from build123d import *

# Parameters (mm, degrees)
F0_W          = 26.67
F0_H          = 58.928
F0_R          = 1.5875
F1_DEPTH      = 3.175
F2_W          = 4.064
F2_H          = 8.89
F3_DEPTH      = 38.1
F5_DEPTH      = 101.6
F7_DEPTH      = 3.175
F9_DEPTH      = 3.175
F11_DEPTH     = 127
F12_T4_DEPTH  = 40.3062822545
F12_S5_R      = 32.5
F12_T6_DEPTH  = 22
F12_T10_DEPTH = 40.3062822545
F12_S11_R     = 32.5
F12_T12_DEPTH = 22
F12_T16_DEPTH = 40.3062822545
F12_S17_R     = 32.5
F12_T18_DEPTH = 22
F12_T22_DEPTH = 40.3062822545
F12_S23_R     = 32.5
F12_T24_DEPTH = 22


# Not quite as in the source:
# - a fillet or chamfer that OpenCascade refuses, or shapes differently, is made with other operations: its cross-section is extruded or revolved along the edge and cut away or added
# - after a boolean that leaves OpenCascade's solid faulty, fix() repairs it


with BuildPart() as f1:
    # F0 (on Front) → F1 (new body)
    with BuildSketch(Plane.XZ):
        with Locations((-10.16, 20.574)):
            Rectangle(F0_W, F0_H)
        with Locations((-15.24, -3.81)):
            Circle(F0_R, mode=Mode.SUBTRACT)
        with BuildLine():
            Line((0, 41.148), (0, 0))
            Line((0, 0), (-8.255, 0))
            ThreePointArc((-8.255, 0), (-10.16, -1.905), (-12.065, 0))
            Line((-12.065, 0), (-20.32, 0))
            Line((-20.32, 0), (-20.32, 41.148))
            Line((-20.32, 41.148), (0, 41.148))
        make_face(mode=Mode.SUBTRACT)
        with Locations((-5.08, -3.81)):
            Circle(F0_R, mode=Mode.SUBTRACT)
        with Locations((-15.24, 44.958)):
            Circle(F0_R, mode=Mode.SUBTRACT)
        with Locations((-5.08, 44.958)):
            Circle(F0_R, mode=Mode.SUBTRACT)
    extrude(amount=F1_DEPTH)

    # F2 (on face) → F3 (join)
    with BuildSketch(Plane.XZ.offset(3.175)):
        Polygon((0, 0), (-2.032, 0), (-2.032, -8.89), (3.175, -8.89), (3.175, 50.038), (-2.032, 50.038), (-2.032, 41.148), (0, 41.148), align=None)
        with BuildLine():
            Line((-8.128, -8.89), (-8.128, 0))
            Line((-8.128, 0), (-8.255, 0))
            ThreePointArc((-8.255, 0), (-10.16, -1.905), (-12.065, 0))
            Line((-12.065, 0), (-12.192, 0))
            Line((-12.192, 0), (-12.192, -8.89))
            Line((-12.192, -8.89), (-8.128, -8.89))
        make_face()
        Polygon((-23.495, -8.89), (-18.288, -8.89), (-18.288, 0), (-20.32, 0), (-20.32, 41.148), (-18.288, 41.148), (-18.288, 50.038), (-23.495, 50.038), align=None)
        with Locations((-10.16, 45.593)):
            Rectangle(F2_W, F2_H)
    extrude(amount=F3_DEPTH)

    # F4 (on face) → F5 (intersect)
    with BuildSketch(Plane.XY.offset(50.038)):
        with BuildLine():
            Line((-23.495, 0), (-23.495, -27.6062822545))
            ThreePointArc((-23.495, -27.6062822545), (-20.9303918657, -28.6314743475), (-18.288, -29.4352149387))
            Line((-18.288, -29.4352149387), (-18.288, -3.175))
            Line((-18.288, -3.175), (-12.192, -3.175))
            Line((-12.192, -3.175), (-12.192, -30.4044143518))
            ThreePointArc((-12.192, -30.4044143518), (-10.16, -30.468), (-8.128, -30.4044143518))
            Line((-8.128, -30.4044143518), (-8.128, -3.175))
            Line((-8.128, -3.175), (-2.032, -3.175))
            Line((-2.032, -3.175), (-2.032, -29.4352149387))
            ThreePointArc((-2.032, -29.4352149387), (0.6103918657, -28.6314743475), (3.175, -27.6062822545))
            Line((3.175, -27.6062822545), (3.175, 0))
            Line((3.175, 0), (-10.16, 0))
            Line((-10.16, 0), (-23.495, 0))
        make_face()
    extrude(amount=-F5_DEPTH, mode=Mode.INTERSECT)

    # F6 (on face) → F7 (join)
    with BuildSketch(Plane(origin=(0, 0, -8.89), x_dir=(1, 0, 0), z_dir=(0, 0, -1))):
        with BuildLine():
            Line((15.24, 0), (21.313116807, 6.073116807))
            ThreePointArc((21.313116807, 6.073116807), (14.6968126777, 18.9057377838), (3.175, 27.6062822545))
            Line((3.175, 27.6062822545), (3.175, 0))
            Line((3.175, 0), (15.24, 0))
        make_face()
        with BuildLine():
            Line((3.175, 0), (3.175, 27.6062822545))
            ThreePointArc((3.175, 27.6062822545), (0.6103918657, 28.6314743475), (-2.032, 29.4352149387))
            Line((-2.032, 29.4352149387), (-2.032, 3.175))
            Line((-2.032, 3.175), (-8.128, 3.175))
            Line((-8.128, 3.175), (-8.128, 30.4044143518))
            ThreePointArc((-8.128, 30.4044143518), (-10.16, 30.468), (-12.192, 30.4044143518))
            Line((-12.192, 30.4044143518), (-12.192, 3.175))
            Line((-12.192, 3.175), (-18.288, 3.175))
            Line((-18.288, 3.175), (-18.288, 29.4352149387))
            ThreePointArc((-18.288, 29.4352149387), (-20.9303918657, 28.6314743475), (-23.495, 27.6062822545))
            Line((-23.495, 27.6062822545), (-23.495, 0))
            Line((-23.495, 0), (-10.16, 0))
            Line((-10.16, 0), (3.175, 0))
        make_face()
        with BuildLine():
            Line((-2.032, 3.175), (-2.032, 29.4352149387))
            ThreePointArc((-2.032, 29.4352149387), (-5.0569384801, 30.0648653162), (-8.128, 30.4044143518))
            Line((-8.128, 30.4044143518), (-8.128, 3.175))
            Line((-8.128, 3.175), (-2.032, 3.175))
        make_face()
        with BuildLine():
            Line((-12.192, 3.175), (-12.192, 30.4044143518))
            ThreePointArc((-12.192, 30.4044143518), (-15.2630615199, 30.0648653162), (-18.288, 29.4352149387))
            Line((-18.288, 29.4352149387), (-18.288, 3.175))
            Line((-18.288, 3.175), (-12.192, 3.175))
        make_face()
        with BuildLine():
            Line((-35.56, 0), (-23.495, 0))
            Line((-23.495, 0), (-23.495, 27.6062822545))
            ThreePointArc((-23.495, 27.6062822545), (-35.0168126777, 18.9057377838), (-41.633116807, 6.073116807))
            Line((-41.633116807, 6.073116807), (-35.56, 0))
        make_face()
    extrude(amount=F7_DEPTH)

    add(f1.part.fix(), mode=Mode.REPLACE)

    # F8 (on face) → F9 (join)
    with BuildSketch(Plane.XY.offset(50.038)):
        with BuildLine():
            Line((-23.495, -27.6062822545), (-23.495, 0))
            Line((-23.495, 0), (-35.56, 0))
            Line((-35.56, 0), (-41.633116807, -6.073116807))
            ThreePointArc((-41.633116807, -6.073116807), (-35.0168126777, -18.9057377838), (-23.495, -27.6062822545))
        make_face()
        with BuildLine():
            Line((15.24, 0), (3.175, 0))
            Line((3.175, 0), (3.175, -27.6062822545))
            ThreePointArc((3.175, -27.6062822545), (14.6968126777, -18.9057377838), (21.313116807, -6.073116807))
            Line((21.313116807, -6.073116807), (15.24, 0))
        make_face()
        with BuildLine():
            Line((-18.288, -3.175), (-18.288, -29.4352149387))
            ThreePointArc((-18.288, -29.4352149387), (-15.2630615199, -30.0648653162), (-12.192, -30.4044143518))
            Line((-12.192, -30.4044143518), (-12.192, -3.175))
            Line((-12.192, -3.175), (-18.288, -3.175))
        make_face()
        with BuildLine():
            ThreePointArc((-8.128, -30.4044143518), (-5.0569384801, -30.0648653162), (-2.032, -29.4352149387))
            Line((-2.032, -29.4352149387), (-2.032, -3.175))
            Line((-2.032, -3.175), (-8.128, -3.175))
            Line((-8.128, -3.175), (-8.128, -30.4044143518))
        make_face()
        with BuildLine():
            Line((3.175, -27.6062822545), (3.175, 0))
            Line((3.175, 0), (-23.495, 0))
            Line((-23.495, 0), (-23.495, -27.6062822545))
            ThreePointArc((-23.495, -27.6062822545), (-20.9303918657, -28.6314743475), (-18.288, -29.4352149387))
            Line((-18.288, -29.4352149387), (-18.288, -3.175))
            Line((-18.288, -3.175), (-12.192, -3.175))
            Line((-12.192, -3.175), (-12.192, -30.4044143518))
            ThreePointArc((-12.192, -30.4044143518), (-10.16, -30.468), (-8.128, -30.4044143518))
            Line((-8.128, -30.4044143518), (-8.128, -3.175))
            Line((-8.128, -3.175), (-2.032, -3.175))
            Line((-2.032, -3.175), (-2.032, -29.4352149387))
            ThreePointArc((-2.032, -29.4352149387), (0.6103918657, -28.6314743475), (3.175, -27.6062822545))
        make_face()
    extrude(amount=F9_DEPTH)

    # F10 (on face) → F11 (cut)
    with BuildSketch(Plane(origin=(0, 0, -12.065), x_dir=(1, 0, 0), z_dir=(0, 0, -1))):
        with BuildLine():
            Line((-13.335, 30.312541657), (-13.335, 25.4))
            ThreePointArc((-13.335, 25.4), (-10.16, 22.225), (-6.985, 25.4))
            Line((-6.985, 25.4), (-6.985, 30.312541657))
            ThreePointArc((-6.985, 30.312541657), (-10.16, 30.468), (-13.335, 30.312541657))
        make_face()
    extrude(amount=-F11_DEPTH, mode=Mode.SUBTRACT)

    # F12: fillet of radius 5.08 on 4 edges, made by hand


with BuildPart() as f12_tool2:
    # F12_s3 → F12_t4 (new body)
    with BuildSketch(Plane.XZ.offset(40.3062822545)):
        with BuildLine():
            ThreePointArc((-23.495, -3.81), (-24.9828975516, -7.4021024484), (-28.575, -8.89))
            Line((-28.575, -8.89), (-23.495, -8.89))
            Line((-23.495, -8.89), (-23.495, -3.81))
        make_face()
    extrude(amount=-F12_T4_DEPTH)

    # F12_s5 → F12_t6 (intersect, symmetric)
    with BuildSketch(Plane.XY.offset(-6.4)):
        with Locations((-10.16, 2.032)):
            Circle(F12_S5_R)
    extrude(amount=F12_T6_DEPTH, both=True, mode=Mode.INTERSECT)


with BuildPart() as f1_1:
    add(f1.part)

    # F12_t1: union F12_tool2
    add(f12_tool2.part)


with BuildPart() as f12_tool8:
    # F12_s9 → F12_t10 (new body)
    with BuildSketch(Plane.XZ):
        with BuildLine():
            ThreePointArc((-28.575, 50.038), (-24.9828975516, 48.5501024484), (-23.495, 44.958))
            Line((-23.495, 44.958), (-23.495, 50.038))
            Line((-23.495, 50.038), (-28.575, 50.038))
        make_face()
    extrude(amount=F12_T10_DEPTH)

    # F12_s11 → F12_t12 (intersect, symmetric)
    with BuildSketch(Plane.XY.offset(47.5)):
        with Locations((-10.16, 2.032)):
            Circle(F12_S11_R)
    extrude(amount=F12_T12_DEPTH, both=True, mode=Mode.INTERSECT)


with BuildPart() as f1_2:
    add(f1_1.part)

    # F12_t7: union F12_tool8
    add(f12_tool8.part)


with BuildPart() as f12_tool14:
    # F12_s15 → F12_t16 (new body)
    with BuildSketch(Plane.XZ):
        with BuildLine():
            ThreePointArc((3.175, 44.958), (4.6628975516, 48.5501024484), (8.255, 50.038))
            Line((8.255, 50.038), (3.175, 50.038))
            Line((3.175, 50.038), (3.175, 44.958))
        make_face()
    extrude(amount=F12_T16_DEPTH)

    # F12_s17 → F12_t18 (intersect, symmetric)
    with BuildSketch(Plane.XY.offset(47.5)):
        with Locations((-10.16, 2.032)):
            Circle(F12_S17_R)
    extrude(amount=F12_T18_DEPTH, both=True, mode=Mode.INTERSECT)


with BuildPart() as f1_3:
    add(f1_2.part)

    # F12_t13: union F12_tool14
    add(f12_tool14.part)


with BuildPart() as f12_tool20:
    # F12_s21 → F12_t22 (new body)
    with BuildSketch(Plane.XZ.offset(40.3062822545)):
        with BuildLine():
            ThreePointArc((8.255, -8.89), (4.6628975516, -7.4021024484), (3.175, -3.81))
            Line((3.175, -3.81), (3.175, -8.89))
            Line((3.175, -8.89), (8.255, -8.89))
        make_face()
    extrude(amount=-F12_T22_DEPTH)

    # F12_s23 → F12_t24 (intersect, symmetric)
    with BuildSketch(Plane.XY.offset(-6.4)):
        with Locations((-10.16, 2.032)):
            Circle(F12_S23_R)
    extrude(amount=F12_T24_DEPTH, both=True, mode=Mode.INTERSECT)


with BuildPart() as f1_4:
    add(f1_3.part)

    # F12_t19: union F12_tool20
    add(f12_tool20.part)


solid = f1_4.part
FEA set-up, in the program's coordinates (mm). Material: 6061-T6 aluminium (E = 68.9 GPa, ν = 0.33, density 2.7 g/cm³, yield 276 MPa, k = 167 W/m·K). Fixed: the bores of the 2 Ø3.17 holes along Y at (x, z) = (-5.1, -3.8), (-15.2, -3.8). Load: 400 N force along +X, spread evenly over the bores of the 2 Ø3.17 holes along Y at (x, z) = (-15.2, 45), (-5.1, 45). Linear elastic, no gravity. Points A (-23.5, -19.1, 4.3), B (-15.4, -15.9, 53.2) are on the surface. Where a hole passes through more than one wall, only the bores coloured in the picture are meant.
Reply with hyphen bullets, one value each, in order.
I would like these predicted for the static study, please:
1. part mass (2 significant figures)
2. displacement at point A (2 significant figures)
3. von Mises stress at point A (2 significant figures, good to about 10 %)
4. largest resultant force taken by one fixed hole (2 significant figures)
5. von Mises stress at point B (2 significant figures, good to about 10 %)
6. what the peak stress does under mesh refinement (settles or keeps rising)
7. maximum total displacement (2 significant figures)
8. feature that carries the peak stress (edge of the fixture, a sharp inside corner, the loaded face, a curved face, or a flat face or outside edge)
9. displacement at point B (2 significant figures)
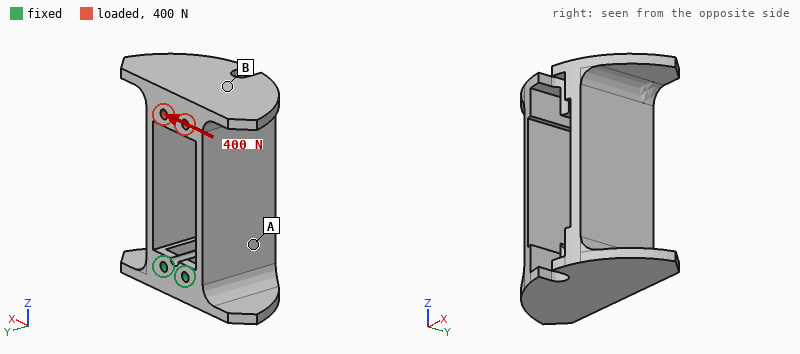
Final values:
- 66 g
- 0.091 mm
- 56 MPa
- 1.3 kN
- 18 MPa
- keeps rising
- 0.58 mm
- edge of the fixture
- 0.50 mm
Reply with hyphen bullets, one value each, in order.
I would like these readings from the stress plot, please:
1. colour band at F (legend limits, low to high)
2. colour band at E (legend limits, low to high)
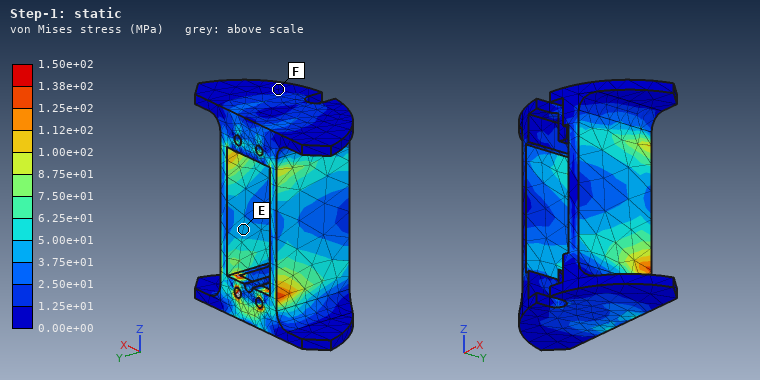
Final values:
- 0.00e+00 to 1.25e+01 MPa
- 3.75e+01 to 5.00e+01 MPa
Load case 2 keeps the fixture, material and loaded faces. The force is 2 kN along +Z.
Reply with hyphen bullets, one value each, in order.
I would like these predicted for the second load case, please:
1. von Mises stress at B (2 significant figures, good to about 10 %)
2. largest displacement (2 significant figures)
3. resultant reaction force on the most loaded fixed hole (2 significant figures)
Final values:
- 14 MPa
- 91 µm
- 1.1 kN
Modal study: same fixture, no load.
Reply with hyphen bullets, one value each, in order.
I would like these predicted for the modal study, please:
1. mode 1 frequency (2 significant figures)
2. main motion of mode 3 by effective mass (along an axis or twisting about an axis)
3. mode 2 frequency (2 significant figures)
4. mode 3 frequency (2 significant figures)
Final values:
- 810 Hz
- twisting about Z
- 820 Hz
- 2100 Hz
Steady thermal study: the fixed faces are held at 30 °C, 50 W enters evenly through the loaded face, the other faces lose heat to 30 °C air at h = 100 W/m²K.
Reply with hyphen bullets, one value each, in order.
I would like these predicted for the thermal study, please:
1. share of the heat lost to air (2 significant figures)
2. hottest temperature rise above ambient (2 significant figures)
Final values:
- 71 %
- 67 K
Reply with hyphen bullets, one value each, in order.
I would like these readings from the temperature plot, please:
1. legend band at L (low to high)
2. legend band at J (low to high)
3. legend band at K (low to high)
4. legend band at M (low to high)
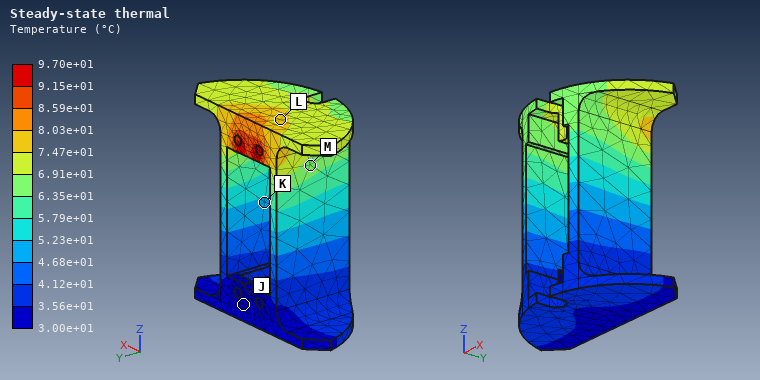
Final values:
- 7.47e+01 to 8.03e+01 °C
- 3.00e+01 to 3.56e+01 °C
- 4.68e+01 to 5.23e+01 °C
- 6.35e+01 to 6.91e+01 °C
